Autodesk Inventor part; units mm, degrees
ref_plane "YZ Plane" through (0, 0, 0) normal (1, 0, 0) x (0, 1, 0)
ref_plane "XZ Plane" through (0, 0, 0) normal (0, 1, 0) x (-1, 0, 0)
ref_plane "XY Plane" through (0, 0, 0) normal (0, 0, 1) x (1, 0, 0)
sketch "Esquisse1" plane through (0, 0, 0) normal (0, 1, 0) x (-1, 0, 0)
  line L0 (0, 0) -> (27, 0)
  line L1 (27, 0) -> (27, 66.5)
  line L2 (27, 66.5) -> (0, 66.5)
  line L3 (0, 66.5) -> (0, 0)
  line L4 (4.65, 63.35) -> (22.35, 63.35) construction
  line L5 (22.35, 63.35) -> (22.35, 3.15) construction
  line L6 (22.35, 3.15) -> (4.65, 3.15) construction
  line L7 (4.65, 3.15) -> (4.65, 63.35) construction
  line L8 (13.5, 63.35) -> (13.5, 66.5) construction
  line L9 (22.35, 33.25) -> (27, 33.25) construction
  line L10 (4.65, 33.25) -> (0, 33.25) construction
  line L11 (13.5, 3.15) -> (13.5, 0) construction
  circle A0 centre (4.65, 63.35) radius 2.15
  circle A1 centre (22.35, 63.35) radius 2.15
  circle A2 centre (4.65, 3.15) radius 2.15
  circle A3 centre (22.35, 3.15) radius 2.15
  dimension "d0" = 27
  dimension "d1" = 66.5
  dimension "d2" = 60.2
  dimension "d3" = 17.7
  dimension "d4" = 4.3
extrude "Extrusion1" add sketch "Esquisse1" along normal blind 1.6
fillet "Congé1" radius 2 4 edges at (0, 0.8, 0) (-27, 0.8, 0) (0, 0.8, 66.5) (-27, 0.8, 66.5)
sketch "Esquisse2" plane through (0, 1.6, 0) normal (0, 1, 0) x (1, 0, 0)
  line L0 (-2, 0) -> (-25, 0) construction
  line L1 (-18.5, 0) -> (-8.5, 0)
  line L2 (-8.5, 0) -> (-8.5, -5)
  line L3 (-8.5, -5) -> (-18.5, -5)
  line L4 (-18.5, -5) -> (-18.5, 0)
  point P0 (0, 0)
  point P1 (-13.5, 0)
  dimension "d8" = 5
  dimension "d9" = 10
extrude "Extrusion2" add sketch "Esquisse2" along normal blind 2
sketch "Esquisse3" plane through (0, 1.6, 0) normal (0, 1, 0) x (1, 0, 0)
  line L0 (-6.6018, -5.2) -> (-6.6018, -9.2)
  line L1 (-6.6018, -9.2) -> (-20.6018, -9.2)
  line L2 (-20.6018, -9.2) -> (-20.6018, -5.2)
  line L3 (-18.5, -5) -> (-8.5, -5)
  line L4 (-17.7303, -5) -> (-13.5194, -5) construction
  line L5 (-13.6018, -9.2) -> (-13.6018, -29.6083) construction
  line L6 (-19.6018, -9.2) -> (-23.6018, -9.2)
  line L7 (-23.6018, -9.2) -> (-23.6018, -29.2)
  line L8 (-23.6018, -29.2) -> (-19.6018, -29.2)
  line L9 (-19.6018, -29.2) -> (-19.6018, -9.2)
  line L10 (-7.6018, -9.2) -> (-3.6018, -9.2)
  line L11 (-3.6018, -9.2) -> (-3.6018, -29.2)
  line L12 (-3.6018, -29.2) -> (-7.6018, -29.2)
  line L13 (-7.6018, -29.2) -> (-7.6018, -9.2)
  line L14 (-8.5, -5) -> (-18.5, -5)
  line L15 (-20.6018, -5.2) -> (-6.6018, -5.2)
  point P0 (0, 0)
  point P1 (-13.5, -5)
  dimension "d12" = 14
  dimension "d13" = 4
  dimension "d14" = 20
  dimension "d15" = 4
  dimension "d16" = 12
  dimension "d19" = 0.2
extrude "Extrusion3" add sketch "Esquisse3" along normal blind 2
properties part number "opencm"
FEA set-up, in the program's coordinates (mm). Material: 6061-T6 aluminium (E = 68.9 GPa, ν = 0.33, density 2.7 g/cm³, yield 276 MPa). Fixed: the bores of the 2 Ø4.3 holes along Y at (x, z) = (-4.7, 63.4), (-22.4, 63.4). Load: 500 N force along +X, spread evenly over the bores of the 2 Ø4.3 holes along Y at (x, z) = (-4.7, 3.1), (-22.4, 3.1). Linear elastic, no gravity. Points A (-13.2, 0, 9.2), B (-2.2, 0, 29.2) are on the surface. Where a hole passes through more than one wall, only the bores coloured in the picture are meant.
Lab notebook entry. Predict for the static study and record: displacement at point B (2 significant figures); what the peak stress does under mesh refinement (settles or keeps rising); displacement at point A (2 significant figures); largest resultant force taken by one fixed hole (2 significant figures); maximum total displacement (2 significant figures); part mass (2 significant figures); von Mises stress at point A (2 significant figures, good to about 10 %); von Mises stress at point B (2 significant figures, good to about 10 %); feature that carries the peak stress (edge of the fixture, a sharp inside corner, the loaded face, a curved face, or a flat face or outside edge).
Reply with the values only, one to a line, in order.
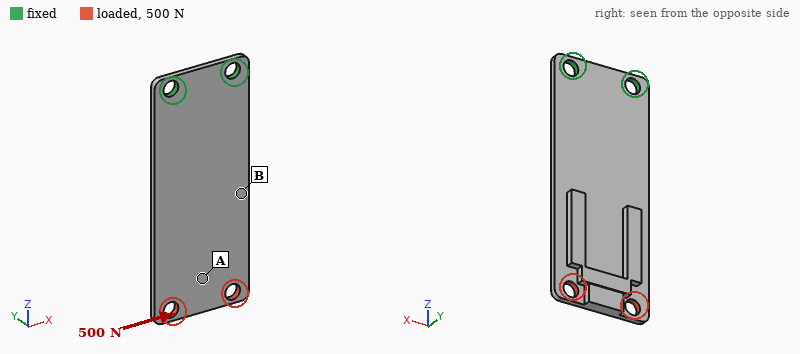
0.11 mm
keeps rising
0.20 mm
1.5 kN
0.26 mm
8.9 g
26 MPa
53 MPa
edge of the fixture
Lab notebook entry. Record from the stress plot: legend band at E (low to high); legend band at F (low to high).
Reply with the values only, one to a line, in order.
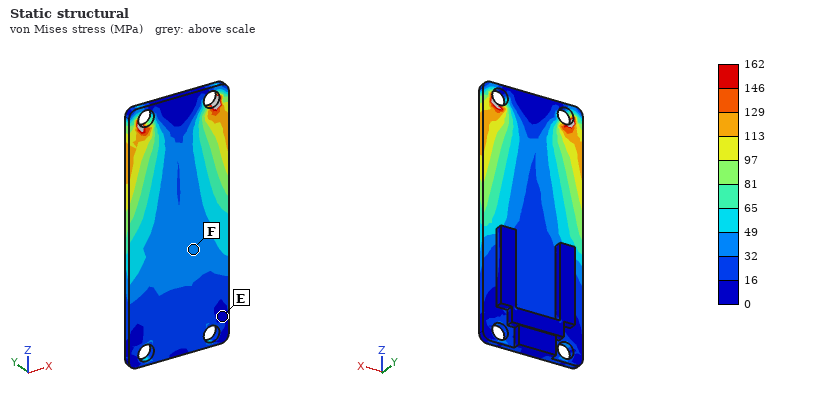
0 to 16 MPa
32 to 49 MPa
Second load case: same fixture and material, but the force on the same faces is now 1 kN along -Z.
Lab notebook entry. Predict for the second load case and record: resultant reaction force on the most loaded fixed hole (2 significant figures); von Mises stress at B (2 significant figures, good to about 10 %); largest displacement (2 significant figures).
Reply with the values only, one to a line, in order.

510 N
26 MPa
61 µm
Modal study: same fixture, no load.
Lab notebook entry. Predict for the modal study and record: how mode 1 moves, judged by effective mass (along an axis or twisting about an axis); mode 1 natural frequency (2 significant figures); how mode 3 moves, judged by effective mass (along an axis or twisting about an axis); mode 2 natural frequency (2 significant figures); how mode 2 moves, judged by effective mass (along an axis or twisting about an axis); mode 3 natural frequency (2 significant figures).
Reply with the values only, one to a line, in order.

along Y
300 Hz
along Y
1700 Hz
twisting about Z
2300 Hz
